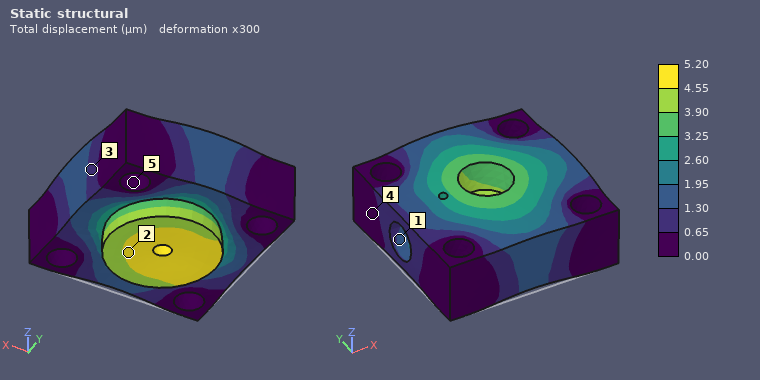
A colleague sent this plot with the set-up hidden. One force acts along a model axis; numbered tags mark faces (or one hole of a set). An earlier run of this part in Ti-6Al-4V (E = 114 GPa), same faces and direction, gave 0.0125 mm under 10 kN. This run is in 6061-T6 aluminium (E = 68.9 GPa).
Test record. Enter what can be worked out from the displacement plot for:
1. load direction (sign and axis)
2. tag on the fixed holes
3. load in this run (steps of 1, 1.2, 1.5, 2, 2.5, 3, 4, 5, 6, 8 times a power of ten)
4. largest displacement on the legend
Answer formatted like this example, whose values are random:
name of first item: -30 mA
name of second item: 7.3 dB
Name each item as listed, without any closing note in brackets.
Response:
load direction: +Z
tag on the fixed holes: 5
load in this run: 2.5 kN
largest displacement on the legend: 5.20 µm
